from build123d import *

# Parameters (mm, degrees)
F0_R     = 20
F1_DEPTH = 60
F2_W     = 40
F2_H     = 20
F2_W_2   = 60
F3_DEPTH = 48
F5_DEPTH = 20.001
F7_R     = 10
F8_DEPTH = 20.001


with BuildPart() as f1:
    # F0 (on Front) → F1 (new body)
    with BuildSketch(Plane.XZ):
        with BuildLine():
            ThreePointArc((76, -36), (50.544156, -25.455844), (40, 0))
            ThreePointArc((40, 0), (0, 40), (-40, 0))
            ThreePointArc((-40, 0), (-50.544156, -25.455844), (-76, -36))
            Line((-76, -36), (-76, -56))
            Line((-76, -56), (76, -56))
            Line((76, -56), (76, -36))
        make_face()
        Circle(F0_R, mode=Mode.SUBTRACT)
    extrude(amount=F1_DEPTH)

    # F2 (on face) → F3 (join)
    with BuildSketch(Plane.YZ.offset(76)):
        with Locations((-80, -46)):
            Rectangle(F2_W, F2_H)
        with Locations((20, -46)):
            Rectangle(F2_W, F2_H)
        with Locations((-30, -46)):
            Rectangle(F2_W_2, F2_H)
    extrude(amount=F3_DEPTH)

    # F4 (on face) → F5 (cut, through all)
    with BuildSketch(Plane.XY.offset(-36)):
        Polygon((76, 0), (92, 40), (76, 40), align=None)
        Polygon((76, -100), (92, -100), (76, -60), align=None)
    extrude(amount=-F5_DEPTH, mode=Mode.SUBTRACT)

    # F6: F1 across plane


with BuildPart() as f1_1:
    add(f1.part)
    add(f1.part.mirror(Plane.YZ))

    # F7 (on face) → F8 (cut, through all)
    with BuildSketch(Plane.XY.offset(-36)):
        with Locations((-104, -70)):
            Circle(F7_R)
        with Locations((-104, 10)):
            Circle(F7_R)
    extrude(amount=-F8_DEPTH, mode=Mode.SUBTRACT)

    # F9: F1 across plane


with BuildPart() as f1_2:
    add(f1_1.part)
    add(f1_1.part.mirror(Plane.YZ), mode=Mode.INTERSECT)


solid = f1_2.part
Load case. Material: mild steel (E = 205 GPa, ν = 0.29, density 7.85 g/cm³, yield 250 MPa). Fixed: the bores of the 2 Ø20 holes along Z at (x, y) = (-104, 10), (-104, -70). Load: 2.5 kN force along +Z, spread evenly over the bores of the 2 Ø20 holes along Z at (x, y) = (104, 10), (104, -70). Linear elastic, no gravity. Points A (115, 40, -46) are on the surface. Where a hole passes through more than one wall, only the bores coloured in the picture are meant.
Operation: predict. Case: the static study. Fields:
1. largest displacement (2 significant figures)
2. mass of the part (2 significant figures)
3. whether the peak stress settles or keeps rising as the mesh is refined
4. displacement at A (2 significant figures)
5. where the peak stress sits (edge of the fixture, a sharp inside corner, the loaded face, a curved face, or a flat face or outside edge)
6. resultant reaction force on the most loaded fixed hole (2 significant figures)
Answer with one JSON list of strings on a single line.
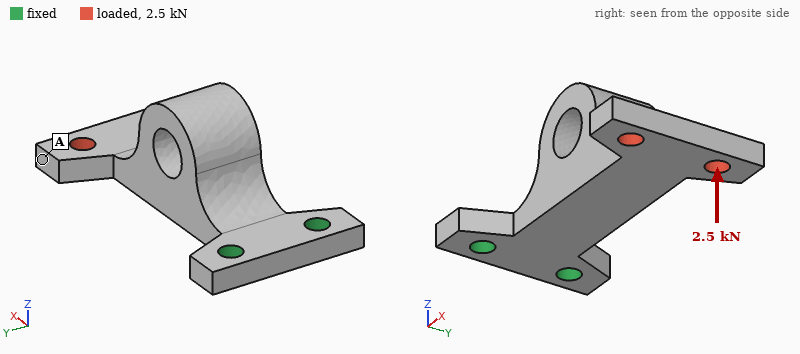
["0.56 mm", "5.4 kg", "keeps rising", "0.53 mm", "a sharp inside corner", "1.3 kN"]
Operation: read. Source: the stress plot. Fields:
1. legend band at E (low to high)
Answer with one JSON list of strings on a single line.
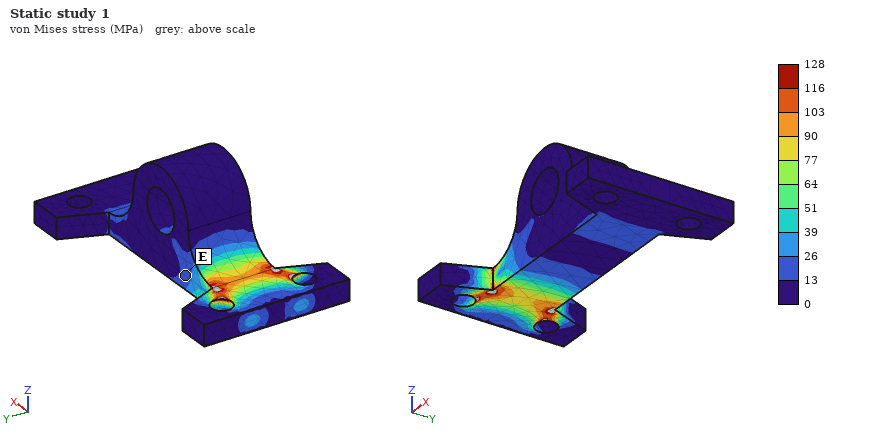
["13 to 26 MPa"]
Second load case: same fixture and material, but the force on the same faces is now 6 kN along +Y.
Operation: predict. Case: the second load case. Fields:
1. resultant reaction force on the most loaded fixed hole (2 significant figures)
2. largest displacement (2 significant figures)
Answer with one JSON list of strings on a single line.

["17 kN", "0.22 mm"]
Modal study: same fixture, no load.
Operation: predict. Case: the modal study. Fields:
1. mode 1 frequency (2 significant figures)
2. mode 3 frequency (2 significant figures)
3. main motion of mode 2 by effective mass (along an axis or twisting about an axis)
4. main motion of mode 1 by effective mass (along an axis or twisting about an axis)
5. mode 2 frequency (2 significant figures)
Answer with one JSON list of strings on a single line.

["270 Hz", "1100 Hz", "along Y", "along Z", "780 Hz"]
